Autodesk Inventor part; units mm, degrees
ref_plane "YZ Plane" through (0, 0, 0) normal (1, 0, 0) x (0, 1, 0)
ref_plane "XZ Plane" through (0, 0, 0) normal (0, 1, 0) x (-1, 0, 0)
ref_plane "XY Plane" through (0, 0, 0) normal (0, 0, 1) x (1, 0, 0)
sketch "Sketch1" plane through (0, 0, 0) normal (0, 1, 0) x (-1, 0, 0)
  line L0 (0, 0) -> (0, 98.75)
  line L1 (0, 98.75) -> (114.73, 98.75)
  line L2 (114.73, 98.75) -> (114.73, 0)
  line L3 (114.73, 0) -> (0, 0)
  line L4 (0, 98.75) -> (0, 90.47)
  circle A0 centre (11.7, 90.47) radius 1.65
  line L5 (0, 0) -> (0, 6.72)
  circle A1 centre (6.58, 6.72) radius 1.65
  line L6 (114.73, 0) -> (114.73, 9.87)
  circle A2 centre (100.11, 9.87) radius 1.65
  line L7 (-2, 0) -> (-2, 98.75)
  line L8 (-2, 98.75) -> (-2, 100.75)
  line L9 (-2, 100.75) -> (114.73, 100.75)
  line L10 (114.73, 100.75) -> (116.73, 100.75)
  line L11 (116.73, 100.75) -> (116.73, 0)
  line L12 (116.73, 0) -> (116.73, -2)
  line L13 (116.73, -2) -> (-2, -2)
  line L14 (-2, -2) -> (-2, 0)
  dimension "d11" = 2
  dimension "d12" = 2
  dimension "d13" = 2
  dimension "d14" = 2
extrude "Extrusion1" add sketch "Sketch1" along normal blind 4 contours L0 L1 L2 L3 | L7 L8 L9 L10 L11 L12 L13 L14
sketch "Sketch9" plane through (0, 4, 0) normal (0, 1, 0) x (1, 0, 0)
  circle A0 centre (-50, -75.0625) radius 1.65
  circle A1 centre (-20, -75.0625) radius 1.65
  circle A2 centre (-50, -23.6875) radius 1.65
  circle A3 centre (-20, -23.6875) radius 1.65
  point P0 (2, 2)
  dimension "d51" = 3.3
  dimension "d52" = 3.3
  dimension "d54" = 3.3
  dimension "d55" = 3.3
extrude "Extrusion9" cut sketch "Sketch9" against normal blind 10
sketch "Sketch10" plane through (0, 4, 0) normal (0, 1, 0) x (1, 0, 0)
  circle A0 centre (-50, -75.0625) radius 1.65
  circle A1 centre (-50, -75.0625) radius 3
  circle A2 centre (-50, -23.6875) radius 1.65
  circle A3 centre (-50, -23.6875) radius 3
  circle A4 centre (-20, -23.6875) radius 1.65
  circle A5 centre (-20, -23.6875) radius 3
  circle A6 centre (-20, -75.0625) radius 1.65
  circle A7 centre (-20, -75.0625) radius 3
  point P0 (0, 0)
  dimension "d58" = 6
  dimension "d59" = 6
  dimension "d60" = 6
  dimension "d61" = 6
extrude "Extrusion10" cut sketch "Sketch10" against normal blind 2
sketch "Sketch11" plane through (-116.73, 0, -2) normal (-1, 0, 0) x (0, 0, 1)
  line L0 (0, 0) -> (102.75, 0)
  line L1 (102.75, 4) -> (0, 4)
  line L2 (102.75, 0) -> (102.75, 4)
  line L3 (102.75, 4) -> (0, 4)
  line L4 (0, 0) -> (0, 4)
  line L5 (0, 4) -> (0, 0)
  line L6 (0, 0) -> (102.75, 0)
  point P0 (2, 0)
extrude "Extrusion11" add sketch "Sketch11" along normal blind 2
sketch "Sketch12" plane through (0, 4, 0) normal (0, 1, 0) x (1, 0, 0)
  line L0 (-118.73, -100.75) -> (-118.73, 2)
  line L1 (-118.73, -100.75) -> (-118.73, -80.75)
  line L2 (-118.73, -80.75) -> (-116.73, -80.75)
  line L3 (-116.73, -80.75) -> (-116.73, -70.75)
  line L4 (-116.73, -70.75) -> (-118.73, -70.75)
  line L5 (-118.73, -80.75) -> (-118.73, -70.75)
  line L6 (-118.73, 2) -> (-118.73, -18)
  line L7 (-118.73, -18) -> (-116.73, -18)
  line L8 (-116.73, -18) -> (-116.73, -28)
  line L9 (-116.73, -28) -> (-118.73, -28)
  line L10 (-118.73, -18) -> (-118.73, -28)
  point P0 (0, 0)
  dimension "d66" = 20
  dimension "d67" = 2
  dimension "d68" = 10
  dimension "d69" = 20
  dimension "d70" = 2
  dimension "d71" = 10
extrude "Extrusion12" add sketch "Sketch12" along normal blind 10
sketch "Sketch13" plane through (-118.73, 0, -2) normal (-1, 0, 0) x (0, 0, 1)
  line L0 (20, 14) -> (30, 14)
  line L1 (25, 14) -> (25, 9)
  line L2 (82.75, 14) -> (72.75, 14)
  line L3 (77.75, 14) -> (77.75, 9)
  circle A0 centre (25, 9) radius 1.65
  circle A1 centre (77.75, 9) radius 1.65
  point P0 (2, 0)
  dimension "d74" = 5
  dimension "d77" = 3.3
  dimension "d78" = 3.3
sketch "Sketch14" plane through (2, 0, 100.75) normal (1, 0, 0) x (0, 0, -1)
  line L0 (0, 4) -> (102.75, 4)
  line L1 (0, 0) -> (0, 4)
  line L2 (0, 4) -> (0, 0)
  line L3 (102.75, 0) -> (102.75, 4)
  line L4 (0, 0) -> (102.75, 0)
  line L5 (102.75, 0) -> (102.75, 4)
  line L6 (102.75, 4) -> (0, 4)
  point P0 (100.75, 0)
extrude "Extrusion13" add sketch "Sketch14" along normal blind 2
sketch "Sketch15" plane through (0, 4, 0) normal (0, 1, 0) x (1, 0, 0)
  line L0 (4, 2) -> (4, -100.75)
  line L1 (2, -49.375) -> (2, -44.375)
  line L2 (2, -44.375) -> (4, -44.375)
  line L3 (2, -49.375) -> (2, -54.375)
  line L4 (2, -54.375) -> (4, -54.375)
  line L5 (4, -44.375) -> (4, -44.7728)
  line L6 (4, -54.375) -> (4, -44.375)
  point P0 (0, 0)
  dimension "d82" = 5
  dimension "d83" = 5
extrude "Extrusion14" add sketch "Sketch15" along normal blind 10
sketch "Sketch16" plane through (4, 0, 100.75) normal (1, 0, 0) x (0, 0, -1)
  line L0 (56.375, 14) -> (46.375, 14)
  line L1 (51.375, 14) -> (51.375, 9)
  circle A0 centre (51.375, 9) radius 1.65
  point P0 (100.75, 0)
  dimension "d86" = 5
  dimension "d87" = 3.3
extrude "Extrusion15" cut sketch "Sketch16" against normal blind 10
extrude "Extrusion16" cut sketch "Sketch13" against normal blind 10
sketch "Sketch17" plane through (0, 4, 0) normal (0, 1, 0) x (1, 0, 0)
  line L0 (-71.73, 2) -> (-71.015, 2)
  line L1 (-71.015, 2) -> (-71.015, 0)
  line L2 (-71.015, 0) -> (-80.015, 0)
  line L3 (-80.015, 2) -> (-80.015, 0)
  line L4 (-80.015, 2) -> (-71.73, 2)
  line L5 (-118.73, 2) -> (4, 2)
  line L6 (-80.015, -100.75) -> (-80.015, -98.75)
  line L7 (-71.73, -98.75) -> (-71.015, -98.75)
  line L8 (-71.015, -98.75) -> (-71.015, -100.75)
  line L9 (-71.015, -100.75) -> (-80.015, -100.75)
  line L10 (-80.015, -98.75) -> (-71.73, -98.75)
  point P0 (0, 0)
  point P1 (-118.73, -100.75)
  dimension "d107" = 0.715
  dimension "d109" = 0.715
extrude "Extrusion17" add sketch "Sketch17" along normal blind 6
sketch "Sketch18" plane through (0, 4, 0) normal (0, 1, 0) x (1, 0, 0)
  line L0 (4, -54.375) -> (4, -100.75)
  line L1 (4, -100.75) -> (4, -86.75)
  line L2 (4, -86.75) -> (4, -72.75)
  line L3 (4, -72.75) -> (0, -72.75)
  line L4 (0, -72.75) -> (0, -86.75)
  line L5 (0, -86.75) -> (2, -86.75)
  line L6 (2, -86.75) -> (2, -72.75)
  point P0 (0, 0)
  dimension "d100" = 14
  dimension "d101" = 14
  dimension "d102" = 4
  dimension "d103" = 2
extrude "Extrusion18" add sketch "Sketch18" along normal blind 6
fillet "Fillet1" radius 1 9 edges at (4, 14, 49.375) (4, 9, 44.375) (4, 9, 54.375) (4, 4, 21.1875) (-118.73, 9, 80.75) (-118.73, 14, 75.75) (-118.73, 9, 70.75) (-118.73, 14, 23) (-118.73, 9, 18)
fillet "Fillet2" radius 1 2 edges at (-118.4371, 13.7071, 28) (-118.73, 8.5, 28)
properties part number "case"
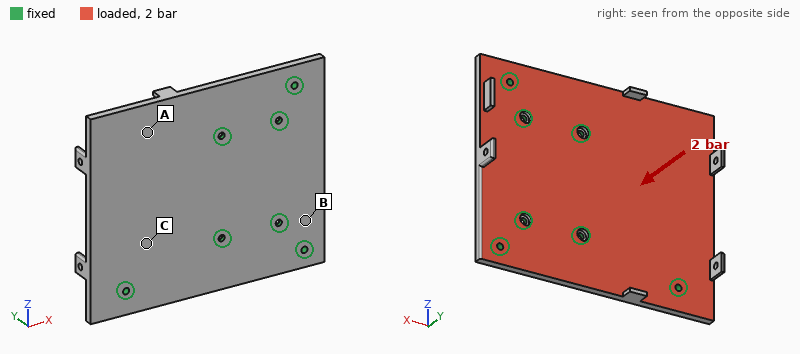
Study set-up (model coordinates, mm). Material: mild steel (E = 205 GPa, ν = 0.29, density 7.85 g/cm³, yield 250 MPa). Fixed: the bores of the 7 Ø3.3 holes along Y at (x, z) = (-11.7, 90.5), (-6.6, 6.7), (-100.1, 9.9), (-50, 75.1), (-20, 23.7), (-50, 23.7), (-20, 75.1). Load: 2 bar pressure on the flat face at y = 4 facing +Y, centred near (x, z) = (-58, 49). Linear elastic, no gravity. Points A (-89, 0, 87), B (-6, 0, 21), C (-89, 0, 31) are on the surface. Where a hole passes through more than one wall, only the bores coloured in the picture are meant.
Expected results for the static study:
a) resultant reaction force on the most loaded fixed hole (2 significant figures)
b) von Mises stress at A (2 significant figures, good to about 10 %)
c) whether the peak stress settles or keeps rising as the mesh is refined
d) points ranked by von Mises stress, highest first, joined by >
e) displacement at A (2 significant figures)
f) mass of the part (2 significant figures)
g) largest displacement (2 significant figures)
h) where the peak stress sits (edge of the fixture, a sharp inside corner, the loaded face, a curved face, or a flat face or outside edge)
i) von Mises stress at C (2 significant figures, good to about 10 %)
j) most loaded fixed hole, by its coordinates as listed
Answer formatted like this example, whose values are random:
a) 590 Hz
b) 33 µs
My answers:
a) 1.4 kN
b) 24 MPa
c) keeps rising
d) C > A > B
e) 0.18 mm
f) 400 g
g) 0.36 mm
h) edge of the fixture
i) 47 MPa
j) (-50, 75.1)
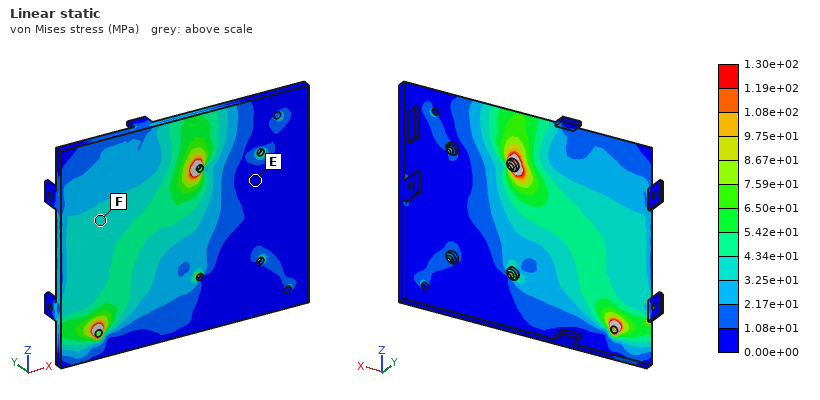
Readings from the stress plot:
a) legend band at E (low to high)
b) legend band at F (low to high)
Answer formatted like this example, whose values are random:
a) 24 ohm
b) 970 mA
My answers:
a) 0.00e+00 to 1.08e+01 MPa
b) 3.25e+01 to 4.34e+01 MPa
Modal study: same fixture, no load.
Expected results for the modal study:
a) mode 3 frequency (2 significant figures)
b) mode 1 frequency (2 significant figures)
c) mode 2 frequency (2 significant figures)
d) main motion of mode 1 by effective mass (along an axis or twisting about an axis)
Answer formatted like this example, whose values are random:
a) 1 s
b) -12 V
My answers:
a) 3700 Hz
b) 920 Hz
c) 2600 Hz
d) along Y
